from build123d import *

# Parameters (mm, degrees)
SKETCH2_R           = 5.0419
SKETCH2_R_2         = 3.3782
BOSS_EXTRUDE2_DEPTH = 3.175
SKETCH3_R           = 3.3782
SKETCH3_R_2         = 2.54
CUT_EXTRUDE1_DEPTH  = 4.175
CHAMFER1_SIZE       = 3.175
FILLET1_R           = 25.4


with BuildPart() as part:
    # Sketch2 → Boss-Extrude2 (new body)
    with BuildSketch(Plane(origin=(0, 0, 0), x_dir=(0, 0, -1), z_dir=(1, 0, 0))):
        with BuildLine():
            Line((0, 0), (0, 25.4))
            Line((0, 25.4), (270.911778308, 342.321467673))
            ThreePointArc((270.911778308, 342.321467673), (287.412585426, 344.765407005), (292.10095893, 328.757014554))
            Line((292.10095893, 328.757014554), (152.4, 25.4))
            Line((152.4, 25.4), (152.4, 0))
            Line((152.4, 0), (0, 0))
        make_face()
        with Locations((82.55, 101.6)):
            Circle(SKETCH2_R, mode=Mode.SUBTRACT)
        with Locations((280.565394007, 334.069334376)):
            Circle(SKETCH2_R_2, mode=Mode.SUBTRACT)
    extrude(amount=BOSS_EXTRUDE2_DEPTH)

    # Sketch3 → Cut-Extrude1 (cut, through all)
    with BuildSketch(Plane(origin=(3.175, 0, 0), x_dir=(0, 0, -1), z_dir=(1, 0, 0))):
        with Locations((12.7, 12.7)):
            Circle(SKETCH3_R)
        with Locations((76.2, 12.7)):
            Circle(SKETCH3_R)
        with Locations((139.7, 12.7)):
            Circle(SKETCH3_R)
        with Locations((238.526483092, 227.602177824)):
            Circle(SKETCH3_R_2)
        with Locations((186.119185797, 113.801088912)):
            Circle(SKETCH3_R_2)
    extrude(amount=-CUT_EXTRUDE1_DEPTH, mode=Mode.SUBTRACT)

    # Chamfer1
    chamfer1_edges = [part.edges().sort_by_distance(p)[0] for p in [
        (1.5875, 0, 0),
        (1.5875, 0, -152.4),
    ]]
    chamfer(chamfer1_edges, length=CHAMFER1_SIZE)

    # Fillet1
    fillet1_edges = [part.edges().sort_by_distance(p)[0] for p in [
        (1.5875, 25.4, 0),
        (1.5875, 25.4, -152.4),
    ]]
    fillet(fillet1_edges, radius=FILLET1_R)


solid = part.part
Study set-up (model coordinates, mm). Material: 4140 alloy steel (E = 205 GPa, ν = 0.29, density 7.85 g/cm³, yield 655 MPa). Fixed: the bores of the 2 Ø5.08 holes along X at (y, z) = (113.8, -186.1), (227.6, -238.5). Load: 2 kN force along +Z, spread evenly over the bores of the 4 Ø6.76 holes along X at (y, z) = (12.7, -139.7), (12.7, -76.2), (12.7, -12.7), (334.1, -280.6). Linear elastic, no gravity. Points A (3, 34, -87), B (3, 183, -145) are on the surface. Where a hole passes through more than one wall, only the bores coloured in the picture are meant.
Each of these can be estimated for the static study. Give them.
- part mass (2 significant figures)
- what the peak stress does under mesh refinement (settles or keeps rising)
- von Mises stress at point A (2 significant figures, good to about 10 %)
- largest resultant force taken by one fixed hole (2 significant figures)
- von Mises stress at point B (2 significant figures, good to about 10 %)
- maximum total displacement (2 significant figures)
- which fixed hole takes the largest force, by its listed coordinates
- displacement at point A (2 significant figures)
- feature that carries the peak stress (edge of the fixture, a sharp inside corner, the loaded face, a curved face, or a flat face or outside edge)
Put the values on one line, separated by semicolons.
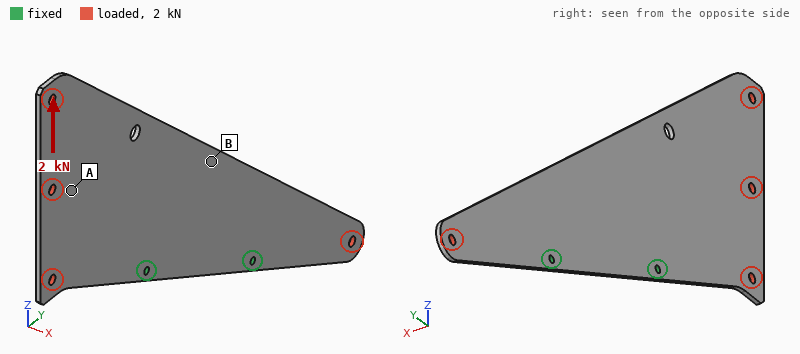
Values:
800 g; keeps rising; 8.7 MPa; 3.2 kN; 22 MPa; 85 µm; (113.8, -186.1); 48 µm; edge of the fixture
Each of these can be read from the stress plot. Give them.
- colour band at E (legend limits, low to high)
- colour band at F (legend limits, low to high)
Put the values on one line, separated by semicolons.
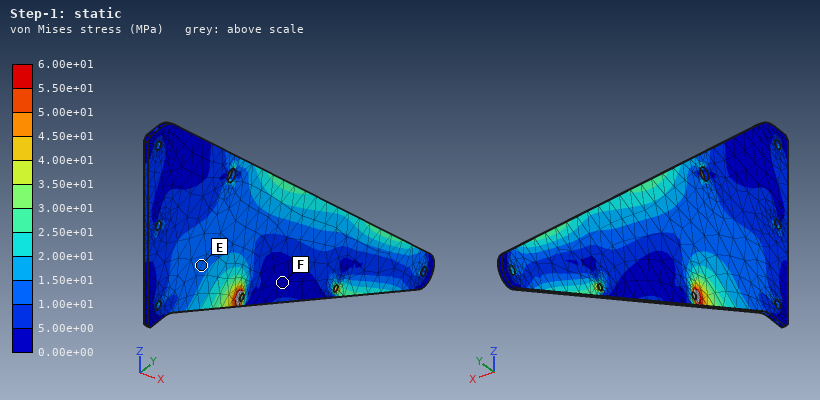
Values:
1.00e+01 to 1.50e+01 MPa; 0.00e+00 to 5.00e+00 MPa
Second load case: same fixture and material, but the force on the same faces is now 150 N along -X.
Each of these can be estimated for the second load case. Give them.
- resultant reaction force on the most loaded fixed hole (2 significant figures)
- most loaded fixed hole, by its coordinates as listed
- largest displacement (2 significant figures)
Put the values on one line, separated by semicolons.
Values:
170 N; (113.8, -186.1); 4.6 mm
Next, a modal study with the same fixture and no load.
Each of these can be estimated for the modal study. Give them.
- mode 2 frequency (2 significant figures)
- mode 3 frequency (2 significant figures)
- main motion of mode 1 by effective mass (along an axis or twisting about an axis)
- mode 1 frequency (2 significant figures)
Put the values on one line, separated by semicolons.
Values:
200 Hz; 220 Hz; along X; 68 Hz
